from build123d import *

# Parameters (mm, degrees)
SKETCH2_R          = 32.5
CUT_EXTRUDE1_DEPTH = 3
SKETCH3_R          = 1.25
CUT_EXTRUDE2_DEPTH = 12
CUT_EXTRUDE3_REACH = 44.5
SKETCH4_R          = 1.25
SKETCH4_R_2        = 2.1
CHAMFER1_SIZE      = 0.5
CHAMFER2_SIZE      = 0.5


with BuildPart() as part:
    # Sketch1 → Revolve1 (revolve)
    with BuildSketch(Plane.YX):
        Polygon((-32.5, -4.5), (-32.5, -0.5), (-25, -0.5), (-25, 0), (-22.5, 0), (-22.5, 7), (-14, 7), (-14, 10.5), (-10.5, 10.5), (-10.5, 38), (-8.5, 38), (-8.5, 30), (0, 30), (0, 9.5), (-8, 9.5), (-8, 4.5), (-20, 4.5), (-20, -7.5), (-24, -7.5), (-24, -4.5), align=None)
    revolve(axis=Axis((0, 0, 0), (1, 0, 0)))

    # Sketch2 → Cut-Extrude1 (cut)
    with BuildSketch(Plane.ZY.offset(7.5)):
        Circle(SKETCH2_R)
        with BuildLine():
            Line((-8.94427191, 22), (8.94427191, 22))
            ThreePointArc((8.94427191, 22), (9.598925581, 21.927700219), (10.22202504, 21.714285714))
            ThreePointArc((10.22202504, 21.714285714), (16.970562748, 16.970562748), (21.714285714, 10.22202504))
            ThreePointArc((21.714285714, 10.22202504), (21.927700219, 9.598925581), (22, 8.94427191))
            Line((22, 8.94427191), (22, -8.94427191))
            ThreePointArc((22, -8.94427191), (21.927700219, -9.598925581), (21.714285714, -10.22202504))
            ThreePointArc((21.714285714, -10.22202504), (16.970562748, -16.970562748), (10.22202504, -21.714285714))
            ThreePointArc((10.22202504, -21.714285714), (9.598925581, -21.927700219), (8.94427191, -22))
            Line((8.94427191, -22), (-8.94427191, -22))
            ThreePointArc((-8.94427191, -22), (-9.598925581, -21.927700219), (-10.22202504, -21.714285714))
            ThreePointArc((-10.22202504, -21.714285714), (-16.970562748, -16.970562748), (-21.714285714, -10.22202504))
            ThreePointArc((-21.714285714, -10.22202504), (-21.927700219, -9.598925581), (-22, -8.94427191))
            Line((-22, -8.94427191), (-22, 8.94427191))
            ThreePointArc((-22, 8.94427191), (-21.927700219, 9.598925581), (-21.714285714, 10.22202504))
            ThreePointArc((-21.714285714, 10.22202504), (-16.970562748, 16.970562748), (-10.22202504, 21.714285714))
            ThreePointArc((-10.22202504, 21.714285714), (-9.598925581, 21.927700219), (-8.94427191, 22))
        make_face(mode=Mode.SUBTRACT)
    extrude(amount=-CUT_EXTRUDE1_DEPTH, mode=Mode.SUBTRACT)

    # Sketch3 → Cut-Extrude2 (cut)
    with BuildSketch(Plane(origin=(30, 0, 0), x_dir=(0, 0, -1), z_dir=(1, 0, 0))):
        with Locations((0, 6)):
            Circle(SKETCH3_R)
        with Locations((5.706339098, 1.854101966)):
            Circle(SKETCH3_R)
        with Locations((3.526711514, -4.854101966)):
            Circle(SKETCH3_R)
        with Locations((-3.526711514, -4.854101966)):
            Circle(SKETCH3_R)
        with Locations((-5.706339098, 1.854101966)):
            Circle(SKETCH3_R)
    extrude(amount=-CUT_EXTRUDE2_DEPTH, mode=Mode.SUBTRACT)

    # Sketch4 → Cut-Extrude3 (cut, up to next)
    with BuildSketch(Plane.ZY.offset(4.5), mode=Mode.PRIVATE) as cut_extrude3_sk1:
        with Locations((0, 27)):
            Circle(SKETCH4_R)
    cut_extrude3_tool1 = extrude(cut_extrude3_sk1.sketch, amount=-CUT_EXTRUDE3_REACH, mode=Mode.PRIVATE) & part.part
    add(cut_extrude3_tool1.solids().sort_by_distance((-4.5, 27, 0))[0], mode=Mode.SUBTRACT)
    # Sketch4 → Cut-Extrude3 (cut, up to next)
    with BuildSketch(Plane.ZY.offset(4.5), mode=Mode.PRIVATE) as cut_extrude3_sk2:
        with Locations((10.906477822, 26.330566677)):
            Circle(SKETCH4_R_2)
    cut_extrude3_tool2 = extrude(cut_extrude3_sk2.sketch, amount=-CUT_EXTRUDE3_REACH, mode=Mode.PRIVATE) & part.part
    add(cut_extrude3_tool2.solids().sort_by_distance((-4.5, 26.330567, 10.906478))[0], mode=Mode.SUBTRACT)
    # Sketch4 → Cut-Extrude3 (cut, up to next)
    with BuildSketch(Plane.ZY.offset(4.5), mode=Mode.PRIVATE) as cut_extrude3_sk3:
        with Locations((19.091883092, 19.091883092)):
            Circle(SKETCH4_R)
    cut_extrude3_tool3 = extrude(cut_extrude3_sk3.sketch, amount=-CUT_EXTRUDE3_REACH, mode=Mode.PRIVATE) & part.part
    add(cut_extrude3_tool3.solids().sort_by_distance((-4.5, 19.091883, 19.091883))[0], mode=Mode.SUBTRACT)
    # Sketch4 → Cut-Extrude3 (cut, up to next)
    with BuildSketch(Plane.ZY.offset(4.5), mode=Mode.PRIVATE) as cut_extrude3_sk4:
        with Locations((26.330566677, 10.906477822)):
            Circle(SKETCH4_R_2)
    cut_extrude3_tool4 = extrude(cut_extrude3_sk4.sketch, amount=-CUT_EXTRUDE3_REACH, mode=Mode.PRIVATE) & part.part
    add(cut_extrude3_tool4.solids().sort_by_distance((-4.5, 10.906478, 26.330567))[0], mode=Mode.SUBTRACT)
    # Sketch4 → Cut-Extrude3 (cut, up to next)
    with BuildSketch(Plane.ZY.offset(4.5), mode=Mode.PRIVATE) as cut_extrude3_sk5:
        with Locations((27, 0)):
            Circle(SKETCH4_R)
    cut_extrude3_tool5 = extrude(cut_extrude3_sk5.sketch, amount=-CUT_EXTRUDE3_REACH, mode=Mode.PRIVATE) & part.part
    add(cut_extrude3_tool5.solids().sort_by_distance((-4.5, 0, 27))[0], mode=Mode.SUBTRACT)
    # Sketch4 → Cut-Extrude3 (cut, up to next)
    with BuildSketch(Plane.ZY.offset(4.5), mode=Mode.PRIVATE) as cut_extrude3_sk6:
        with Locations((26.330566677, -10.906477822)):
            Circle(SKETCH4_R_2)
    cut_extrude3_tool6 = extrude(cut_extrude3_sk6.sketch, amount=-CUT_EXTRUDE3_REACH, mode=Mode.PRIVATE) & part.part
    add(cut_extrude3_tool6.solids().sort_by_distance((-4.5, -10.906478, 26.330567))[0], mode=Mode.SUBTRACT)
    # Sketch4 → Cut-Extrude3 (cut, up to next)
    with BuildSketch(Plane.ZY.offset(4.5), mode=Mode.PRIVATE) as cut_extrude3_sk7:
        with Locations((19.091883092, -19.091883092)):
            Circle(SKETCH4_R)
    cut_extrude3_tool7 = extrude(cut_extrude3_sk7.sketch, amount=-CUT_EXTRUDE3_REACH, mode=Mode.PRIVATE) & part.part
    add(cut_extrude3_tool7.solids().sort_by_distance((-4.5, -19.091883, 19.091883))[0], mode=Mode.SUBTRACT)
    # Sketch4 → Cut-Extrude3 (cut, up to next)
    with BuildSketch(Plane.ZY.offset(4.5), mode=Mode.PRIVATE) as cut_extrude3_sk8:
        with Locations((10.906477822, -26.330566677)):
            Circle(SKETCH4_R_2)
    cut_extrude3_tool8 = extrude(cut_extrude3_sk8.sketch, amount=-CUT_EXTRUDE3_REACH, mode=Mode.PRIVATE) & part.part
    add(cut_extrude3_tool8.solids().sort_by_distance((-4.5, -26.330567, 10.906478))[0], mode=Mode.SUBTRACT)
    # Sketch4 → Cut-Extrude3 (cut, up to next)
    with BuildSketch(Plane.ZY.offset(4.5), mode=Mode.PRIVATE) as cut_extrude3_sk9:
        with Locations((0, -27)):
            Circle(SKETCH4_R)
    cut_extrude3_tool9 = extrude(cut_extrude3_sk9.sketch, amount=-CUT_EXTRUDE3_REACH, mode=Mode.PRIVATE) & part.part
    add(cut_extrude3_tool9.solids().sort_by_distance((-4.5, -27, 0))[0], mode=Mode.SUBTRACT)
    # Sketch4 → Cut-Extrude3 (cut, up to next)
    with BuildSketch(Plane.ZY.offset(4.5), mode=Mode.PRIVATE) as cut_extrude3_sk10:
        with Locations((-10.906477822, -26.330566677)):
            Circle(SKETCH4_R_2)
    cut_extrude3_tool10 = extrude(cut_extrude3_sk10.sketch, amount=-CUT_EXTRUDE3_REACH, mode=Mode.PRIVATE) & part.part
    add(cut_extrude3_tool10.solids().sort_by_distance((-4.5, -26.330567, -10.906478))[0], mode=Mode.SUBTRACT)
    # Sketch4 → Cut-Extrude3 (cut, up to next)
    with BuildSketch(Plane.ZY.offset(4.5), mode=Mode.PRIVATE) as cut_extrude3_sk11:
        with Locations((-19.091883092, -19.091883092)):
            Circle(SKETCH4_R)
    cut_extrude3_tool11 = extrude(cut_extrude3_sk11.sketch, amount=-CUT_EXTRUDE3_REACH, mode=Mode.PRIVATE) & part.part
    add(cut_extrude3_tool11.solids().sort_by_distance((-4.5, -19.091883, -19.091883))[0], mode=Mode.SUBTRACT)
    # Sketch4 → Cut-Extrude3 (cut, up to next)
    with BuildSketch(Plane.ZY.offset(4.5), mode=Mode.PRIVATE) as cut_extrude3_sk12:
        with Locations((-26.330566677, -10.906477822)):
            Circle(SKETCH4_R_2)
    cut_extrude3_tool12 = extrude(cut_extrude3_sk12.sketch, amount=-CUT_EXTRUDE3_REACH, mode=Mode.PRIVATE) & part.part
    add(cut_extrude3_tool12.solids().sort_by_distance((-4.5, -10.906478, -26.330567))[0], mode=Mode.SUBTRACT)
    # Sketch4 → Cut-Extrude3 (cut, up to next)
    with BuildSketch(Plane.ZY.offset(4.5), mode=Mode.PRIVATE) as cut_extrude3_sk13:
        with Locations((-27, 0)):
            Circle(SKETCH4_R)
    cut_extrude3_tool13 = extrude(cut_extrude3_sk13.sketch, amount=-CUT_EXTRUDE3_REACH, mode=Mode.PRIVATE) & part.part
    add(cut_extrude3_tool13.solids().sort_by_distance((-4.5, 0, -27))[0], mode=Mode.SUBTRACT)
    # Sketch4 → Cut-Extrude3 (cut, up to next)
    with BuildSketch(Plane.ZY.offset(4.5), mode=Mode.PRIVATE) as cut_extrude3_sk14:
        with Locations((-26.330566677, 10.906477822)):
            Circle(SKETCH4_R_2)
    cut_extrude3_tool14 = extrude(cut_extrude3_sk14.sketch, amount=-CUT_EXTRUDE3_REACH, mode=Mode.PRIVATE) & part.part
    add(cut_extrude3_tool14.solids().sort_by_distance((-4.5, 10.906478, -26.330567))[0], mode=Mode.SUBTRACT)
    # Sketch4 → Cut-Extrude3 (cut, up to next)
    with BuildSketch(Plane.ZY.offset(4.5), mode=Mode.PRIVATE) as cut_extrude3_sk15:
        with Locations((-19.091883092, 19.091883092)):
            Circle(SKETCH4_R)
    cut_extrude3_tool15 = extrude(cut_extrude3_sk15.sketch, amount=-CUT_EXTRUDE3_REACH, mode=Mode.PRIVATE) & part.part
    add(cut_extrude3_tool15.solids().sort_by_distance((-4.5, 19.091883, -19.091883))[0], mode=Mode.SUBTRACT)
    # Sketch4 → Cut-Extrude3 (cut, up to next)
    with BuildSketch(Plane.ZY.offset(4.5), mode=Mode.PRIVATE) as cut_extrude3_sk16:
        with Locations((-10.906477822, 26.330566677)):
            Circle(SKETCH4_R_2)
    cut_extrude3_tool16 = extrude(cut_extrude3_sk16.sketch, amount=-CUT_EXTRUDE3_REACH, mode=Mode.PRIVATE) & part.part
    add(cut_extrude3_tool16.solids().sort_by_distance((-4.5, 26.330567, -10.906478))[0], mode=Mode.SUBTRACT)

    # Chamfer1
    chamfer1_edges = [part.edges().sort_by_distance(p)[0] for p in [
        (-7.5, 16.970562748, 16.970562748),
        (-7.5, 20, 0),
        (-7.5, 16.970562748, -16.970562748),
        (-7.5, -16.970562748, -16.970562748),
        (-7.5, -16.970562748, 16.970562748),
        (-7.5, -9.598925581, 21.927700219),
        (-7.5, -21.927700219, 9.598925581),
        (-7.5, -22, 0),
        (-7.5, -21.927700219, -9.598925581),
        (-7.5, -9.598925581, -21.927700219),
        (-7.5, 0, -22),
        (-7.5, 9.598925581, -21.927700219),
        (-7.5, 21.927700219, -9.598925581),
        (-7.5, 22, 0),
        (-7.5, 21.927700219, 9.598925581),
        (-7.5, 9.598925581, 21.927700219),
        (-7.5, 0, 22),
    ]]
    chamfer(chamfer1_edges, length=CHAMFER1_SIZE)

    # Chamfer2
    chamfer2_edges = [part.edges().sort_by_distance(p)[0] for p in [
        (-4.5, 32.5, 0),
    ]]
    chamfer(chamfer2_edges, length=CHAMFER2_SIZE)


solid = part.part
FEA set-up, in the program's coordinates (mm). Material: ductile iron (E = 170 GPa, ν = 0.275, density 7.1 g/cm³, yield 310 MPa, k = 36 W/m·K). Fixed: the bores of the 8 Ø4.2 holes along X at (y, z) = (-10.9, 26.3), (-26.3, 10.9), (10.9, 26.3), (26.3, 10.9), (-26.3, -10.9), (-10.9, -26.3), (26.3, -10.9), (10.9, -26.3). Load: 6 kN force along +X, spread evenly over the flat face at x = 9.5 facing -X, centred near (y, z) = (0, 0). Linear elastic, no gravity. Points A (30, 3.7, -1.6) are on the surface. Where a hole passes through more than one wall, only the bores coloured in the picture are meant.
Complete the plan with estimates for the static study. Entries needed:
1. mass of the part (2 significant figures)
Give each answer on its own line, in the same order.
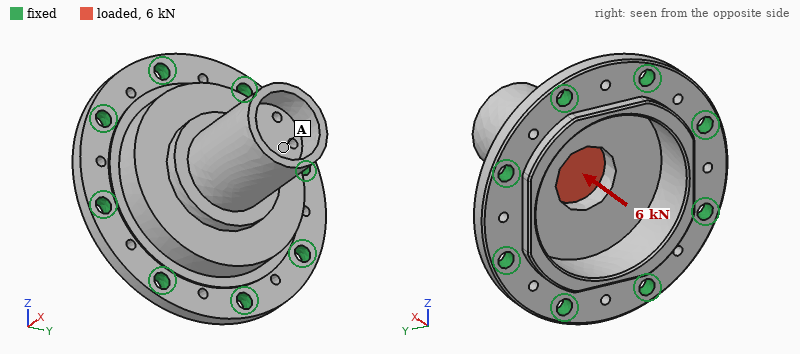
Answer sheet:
170 g
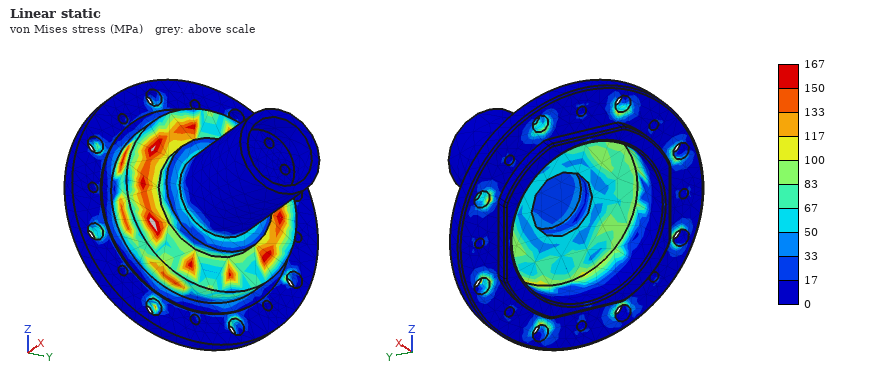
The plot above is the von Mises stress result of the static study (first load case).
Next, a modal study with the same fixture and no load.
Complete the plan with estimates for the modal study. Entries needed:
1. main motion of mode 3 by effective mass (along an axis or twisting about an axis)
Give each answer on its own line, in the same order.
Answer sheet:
along X
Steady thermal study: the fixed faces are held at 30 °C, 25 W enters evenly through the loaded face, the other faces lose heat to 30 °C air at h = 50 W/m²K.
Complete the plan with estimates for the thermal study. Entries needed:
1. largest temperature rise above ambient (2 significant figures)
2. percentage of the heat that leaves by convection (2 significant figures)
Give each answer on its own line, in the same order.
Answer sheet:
54 K
42 %
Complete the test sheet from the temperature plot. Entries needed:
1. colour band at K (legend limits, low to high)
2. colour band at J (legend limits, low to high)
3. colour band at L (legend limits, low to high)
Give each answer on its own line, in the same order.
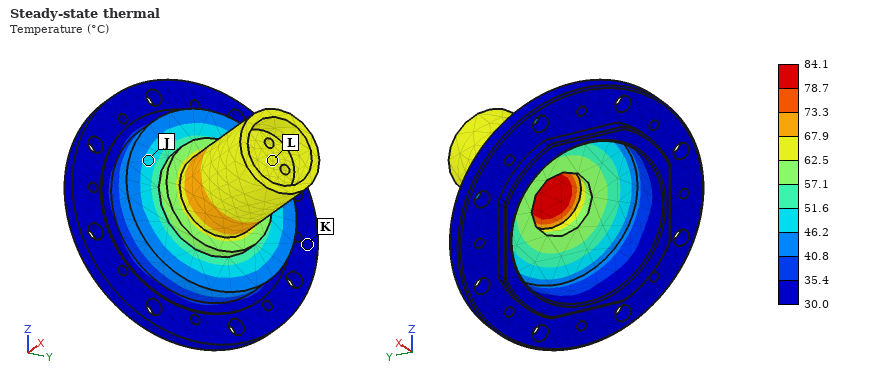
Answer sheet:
30.0 to 35.4 °C
46.2 to 51.6 °C
62.5 to 67.9 °C
